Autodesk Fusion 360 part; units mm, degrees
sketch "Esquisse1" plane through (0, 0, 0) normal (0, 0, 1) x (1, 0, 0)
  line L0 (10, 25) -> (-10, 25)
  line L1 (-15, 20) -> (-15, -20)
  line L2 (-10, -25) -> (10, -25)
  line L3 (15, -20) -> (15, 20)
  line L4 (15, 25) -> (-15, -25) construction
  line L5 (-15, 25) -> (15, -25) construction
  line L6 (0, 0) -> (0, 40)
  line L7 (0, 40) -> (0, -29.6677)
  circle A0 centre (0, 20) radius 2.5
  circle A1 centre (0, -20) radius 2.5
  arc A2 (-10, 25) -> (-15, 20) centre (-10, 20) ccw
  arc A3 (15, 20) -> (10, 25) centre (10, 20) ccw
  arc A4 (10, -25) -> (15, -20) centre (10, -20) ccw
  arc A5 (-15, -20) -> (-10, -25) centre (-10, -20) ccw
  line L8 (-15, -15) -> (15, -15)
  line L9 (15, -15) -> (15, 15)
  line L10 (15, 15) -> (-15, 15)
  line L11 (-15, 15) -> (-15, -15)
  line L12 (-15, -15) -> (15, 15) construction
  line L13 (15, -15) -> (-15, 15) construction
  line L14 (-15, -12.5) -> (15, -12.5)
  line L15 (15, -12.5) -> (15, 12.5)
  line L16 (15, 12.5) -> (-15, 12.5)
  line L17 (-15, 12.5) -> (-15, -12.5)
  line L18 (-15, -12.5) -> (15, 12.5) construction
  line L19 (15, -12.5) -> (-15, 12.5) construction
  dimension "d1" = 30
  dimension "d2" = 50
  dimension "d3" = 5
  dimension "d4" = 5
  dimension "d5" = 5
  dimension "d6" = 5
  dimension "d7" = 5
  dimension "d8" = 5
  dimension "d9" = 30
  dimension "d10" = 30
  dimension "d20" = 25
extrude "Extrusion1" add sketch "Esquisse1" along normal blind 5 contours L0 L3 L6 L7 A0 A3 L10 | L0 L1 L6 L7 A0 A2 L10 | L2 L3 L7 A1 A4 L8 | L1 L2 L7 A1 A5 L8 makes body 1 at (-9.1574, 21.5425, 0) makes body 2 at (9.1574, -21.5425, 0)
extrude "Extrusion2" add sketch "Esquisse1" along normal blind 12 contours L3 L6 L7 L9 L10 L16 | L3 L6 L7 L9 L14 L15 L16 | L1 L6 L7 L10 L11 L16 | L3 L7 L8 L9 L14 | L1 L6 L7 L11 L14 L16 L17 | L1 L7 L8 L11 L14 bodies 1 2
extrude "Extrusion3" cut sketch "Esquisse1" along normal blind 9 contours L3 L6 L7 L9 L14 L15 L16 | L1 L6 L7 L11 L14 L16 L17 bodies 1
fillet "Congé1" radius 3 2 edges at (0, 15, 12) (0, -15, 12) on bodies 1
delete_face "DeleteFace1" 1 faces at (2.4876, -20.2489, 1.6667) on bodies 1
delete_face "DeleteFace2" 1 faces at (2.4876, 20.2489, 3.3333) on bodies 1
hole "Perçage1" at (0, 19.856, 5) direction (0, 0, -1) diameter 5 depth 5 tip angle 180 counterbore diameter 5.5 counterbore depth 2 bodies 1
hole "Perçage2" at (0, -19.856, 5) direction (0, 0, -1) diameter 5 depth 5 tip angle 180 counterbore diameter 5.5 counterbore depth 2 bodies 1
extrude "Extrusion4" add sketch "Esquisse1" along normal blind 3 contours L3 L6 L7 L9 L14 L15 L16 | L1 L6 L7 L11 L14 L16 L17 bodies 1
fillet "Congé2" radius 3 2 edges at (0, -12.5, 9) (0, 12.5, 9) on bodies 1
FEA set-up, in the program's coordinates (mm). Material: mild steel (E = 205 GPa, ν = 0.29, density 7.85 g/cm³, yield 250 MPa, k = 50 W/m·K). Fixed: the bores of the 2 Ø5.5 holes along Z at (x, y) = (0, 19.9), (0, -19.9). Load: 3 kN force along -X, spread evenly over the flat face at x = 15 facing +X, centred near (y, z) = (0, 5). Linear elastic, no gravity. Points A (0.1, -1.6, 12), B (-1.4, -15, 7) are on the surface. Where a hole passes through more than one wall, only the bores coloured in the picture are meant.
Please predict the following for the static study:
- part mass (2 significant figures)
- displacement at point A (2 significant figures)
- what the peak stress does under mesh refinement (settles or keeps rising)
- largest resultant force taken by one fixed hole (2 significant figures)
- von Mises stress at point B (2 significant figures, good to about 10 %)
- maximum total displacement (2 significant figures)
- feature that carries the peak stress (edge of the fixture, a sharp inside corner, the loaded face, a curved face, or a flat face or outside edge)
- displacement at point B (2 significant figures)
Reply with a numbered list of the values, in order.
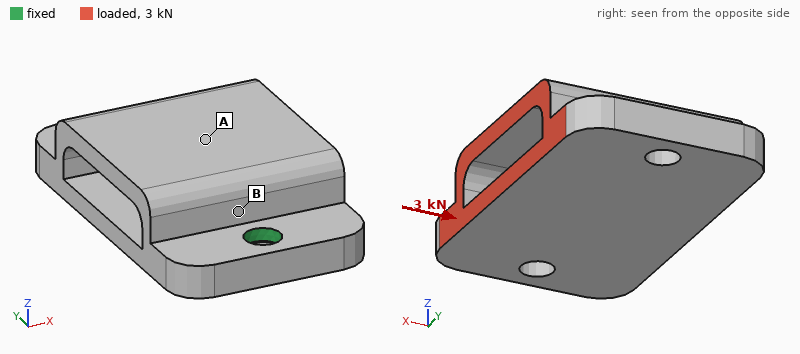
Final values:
1. 70 g
2. 5.6 µm
3. keeps rising
4. 1.5 kN
5. 27 MPa
6. 8.9 µm
7. edge of the fixture
8. 2.8 µm
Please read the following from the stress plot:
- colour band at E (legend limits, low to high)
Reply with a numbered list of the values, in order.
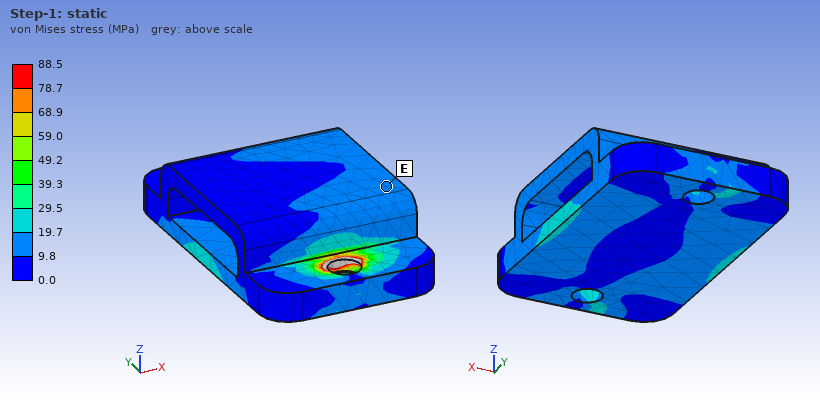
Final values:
1. 9.8 to 19.7 MPa
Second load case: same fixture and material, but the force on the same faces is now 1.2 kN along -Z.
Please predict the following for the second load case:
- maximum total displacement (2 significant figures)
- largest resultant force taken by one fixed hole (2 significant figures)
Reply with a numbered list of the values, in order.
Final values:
1. 35 µm
2. 600 N
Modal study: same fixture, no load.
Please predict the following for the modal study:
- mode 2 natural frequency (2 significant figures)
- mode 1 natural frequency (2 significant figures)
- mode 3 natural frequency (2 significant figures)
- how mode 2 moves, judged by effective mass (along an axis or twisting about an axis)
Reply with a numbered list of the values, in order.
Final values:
1. 13 kHz
2. 7500 Hz
3. 15 kHz
4. along Z
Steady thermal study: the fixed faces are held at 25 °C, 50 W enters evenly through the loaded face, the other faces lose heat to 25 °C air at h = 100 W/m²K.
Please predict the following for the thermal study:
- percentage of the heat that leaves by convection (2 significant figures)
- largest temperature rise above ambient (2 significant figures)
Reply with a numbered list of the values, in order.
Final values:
1. 32 %
2. 74 K
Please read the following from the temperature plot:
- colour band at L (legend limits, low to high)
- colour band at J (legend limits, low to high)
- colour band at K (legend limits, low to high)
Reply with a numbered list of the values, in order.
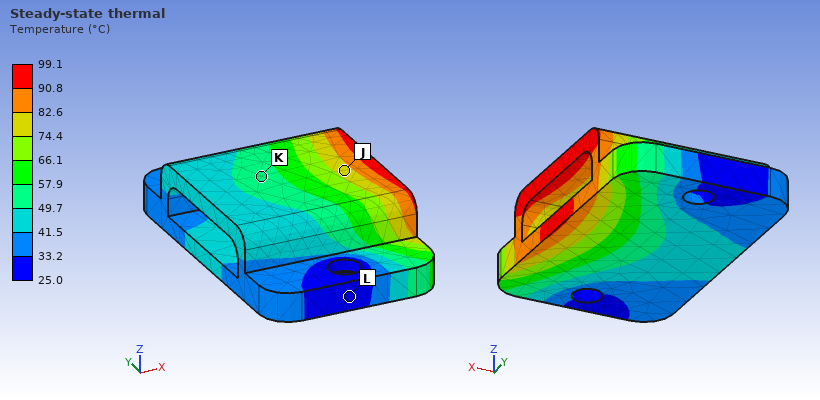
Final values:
1. 25.0 to 33.2 °C
2. 74.4 to 82.6 °C
3. 49.7 to 57.9 °C
